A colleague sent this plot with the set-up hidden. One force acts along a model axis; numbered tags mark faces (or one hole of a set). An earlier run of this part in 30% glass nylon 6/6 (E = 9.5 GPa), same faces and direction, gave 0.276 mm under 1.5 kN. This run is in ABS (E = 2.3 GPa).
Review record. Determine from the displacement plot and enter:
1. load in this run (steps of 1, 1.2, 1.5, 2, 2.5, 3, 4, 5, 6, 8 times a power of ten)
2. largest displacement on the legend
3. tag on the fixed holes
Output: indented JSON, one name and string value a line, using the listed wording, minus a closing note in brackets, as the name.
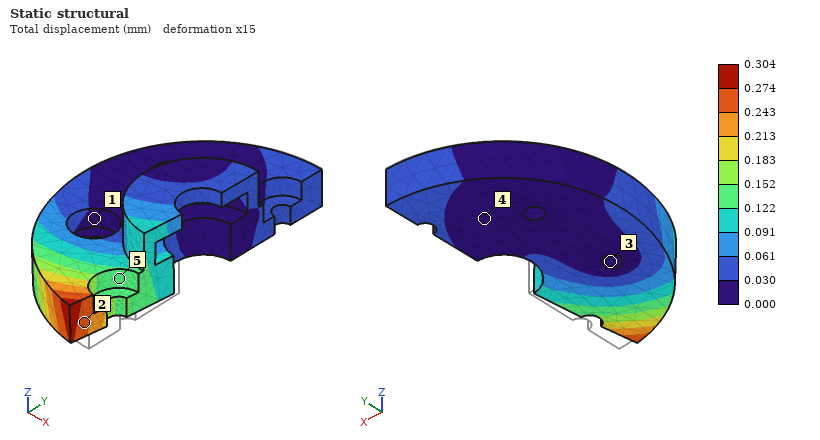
{
  "load in this run": "400 N",
  "largest displacement on the legend": "0.304 mm",
  "tag on the fixed holes": "3"
}
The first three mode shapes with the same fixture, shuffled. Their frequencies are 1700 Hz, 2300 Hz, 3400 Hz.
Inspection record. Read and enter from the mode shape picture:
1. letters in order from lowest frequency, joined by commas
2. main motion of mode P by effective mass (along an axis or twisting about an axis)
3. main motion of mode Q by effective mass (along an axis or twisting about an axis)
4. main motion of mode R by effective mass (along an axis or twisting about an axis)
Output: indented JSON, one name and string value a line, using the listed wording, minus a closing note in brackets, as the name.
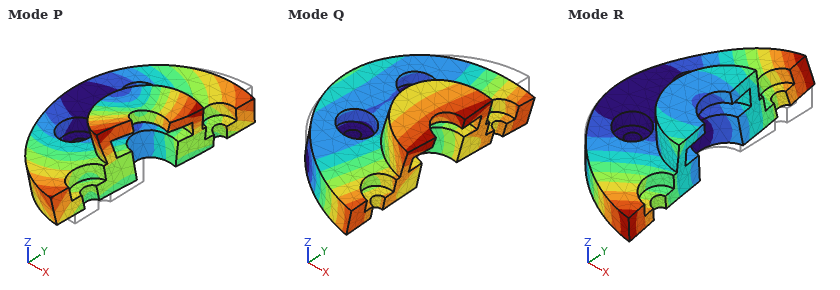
{
  "letters in order from lowest frequency, joined by commas": "Q, R, P",
  "main motion of mode P by effective mass": "along Y",
  "main motion of mode Q by effective mass": "along Z",
  "main motion of mode R by effective mass": "twisting about X"
}
